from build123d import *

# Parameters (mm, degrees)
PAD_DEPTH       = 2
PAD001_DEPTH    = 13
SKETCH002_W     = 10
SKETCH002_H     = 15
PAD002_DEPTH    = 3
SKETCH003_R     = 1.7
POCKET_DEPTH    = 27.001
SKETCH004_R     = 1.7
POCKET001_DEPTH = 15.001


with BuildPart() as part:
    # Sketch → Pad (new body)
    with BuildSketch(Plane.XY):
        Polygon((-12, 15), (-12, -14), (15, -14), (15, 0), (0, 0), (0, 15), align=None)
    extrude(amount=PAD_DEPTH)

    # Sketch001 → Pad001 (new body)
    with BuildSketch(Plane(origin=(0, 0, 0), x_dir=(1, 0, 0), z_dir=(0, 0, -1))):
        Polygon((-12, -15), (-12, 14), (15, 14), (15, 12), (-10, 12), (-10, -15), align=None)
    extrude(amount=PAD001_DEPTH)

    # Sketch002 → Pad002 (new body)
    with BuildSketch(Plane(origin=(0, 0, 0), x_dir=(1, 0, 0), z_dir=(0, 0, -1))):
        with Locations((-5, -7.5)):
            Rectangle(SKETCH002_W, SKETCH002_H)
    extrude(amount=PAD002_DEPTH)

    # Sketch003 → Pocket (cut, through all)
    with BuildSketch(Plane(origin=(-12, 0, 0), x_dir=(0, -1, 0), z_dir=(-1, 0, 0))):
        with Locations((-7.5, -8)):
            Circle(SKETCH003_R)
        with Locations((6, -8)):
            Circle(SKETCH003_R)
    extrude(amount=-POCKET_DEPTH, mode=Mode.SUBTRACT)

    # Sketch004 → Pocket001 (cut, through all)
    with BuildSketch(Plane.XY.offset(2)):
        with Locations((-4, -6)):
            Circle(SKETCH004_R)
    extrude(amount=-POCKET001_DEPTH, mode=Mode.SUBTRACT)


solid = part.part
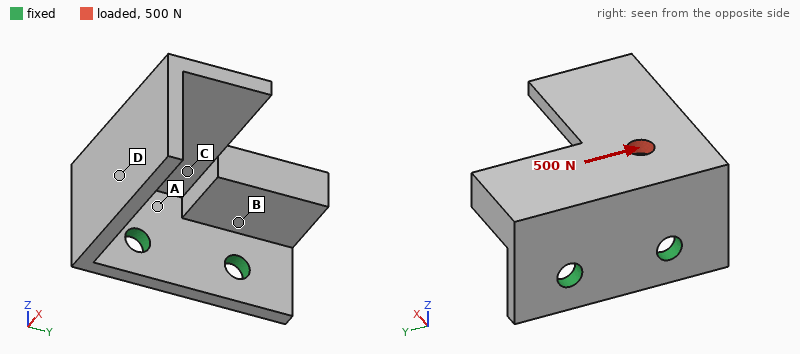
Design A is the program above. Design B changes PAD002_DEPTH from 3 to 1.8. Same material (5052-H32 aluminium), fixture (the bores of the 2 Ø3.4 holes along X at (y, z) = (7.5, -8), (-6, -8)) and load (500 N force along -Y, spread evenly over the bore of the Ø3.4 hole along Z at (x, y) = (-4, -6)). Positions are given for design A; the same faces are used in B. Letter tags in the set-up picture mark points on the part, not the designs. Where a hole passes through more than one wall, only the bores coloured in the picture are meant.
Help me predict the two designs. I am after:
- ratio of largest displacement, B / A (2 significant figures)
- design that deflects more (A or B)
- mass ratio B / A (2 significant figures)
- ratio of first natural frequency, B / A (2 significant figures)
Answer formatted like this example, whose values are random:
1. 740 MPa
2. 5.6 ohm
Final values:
1. 1.2
2. B
3. 0.94
4. 0.97
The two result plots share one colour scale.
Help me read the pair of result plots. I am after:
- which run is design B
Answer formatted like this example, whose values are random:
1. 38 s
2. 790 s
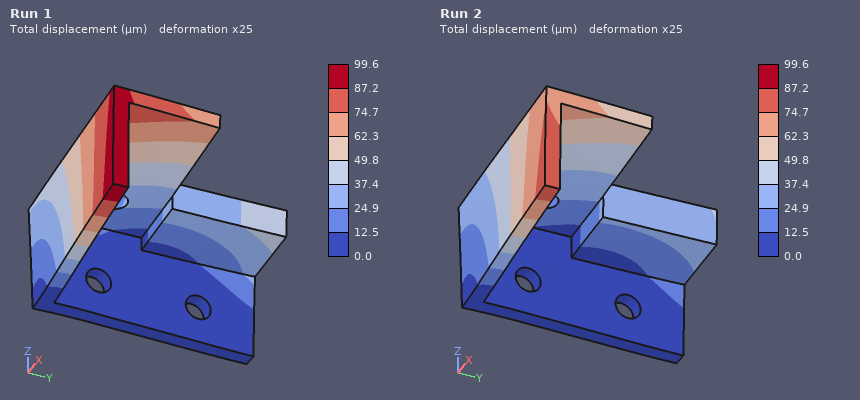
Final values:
1. Run 1
